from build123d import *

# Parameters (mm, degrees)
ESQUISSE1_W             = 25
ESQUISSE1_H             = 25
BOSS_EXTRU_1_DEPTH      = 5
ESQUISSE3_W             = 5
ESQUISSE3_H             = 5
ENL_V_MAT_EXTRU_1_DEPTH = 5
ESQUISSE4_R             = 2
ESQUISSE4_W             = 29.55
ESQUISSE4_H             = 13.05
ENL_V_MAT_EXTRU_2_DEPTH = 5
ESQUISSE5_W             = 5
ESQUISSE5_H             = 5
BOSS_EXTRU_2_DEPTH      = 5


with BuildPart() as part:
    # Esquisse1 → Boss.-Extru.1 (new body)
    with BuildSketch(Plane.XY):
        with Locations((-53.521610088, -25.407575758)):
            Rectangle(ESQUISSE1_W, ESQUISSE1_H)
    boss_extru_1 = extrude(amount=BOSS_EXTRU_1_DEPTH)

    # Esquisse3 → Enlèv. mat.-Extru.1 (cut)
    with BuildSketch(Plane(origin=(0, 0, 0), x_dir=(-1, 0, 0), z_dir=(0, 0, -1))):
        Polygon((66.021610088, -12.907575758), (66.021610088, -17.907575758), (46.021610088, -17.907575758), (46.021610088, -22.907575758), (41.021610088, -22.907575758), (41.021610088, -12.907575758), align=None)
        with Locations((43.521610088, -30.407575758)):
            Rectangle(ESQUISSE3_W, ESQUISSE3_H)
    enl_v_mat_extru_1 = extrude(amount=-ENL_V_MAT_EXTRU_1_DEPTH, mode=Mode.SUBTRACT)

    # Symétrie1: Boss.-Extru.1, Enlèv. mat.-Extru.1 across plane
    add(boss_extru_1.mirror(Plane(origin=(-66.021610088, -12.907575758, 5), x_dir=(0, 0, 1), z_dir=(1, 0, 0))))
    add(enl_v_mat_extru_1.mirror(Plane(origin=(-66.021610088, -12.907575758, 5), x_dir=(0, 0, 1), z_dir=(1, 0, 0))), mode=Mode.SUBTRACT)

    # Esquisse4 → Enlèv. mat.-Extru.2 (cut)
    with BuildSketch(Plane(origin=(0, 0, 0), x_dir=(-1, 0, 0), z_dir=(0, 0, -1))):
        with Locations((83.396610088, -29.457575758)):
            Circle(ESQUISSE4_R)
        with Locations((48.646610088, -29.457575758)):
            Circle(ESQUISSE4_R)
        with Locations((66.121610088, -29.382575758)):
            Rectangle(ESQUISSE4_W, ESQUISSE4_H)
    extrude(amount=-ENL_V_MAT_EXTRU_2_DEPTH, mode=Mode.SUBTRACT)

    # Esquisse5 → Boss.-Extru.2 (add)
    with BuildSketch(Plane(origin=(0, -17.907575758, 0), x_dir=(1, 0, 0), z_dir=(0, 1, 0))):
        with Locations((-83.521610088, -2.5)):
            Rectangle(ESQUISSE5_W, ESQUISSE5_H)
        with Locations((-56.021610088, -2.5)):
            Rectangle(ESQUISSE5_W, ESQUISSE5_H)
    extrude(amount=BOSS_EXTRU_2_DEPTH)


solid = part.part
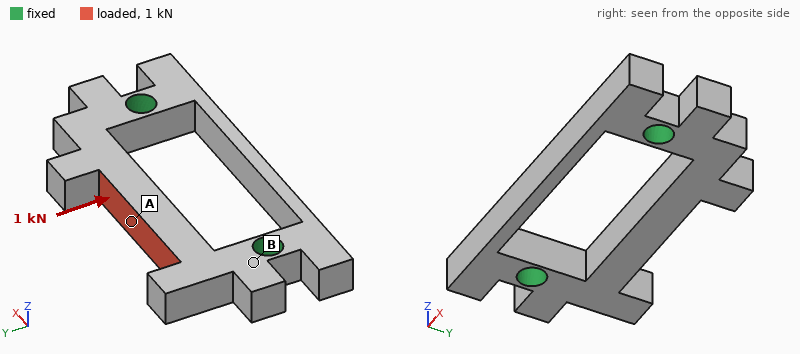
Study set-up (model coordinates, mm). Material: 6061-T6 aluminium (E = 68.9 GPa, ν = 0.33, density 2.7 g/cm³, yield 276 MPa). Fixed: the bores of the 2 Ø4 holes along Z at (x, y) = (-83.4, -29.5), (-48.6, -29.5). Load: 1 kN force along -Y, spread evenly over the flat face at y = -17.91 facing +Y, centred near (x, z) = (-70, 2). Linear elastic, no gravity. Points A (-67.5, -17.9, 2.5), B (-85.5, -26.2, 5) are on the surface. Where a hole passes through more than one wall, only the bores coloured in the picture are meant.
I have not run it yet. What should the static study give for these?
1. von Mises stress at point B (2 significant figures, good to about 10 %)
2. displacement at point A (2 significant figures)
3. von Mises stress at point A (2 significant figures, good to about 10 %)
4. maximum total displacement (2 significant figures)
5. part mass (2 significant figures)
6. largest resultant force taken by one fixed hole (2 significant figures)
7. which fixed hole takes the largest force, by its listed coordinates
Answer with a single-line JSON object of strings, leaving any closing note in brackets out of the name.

{"von Mises stress at point B": "24 MPa", "displacement at point A": "58 µm", "von Mises stress at point A": "120 MPa", "maximum total displacement": "59 µm", "part mass": "7.3 g", "largest resultant force taken by one fixed hole": "760 N", "which fixed hole takes the largest force, by its listed coordinates": "(-83.4, -29.5)"}
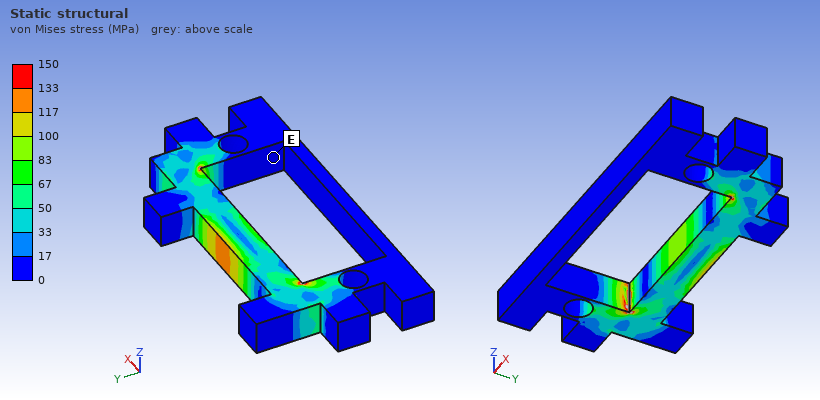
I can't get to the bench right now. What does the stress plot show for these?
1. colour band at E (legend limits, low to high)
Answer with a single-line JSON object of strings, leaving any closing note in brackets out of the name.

{"colour band at E": "0 to 17 MPa"}
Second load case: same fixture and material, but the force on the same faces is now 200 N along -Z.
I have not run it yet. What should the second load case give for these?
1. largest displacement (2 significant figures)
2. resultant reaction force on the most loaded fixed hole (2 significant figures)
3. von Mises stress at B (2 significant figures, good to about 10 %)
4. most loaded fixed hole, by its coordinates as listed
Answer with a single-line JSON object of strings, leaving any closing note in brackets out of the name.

{"largest displacement": "30 µm", "resultant reaction force on the most loaded fixed hole": "120 N", "von Mises stress at B": "30 MPa", "most loaded fixed hole, by its coordinates as listed": "(-83.4, -29.5)"}
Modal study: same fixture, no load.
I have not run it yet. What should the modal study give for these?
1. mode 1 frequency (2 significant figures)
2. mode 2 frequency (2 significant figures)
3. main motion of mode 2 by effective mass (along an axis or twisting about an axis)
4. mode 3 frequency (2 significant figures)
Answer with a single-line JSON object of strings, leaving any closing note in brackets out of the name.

{"mode 1 frequency": "10000 Hz", "mode 2 frequency": "11 kHz", "main motion of mode 2 by effective mass": "along Z", "mode 3 frequency": "16 kHz"}
